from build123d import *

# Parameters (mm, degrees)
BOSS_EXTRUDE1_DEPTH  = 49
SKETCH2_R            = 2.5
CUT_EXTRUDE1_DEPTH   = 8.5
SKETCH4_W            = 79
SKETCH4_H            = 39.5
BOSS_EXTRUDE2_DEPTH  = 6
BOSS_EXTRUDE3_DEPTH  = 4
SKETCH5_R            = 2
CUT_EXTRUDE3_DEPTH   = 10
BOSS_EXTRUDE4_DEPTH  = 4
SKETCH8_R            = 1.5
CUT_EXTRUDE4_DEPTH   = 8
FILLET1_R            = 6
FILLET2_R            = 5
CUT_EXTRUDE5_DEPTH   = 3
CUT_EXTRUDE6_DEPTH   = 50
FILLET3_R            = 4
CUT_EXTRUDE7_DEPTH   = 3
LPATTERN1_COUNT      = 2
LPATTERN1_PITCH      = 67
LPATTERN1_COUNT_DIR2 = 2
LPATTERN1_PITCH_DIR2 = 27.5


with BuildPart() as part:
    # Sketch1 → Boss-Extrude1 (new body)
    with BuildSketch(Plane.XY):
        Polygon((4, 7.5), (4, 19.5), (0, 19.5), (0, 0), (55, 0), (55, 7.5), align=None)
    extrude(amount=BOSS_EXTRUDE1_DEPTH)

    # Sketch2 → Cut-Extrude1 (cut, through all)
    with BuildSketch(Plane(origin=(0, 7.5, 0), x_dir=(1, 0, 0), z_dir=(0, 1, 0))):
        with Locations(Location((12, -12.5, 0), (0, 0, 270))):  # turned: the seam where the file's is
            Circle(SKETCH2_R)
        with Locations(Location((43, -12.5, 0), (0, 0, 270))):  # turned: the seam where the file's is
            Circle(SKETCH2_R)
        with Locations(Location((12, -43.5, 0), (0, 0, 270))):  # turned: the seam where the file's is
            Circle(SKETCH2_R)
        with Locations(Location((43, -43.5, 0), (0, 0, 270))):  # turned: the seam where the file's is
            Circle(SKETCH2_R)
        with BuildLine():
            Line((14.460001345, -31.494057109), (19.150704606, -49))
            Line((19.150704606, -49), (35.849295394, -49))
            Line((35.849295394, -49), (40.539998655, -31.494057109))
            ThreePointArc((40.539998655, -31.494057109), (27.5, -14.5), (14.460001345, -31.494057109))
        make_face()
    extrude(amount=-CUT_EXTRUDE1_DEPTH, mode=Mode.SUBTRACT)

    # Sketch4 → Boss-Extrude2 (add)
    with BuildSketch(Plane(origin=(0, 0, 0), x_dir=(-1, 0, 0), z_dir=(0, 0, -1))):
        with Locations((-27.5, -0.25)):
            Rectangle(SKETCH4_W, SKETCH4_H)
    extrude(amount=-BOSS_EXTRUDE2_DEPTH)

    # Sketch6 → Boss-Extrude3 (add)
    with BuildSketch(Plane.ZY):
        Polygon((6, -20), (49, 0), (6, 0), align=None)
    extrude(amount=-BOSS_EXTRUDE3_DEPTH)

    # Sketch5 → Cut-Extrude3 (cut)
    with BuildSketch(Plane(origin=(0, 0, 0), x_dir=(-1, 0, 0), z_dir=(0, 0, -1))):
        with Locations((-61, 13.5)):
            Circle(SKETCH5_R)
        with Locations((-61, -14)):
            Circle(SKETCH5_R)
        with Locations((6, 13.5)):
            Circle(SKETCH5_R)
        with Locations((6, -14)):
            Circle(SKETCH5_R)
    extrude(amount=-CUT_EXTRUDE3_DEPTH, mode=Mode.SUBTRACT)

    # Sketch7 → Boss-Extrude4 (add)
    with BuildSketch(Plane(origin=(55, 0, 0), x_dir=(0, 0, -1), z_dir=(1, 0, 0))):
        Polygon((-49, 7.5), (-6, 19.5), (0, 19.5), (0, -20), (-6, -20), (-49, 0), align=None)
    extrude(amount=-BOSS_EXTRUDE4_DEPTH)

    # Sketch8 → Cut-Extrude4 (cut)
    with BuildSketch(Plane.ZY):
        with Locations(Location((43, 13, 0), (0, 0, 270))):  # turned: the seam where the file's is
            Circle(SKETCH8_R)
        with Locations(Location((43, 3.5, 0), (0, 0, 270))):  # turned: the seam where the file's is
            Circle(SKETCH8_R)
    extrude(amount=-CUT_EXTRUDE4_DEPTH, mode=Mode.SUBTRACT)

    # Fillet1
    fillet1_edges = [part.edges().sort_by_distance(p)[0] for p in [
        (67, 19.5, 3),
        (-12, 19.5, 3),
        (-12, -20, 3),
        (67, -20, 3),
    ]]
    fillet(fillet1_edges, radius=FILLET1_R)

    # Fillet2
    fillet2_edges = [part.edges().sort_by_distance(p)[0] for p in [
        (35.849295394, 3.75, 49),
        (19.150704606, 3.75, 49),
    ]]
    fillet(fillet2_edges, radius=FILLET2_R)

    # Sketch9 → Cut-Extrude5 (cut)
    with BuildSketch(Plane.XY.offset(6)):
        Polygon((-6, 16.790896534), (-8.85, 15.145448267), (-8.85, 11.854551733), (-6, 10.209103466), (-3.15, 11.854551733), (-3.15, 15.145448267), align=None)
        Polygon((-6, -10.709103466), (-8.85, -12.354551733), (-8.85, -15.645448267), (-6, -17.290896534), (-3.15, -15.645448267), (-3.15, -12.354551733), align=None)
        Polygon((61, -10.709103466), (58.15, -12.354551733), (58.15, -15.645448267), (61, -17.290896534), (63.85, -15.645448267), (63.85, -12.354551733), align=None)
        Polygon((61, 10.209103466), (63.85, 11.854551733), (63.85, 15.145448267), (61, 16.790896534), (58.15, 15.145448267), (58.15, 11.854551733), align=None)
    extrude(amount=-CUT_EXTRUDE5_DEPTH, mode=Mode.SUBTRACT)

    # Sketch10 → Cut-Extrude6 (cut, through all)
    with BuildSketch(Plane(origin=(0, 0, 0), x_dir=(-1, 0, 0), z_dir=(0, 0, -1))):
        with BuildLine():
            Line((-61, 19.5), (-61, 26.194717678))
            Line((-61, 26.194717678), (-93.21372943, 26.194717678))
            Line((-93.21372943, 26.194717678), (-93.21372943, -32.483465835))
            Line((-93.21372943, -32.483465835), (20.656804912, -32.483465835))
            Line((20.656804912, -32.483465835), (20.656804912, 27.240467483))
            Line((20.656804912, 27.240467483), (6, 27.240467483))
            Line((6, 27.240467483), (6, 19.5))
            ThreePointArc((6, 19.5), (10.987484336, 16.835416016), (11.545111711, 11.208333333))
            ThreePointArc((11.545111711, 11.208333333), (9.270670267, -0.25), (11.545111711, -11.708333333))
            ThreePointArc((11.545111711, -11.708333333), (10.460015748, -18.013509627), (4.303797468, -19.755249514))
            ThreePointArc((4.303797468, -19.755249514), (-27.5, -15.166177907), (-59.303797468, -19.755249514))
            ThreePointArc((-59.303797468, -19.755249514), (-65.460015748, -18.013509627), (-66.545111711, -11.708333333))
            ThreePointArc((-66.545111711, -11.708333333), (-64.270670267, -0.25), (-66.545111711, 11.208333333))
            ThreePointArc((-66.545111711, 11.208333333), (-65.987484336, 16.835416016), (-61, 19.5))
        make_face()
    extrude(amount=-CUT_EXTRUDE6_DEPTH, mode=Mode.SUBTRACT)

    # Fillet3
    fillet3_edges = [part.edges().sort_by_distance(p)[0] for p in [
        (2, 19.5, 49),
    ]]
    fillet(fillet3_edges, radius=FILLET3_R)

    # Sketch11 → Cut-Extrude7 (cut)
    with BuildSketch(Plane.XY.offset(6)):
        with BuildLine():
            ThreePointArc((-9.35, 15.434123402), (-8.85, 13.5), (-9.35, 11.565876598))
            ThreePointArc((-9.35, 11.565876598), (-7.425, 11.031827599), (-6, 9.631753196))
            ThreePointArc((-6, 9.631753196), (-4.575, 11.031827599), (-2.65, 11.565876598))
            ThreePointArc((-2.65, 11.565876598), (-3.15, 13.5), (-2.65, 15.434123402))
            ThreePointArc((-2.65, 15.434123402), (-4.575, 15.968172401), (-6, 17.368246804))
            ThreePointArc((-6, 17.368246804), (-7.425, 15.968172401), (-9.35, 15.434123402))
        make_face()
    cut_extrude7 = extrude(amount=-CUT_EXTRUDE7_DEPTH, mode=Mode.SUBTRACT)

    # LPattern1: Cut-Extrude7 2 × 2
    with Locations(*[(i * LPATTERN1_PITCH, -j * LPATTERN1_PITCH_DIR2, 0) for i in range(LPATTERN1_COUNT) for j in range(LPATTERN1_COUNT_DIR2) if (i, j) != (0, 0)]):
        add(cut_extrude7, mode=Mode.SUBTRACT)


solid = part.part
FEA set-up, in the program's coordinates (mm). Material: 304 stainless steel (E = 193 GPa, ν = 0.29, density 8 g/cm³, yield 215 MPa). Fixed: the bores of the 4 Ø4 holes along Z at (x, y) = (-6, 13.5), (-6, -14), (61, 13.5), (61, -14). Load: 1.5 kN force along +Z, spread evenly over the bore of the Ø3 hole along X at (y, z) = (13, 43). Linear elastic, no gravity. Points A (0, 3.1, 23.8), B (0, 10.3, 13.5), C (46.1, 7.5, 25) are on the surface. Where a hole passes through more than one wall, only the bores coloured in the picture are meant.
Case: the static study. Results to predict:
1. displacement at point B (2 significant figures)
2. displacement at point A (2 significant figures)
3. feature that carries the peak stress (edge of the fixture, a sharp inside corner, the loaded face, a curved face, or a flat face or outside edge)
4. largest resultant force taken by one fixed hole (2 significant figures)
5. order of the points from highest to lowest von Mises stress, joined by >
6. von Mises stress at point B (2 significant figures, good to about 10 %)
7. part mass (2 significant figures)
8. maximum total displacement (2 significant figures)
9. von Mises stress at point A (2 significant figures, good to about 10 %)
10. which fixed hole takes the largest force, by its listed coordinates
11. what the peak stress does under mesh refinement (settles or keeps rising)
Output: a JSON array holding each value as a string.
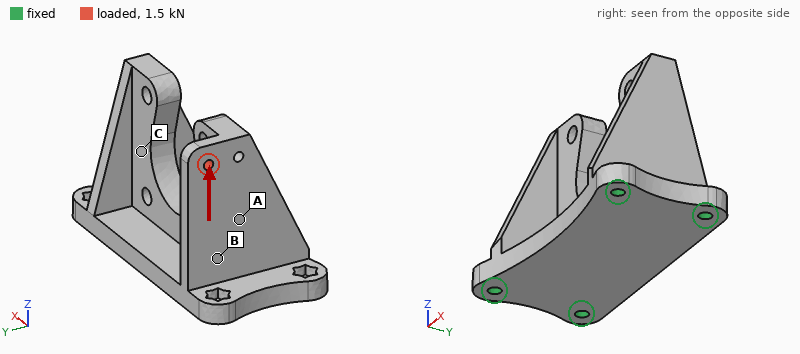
["5.9 µm", "6.3 µm", "edge of the fixture", "1.4 kN", "B > A > C", "25 MPa", "270 g", "18 µm", "11 MPa", "(-6, 13.5)", "keeps rising"]
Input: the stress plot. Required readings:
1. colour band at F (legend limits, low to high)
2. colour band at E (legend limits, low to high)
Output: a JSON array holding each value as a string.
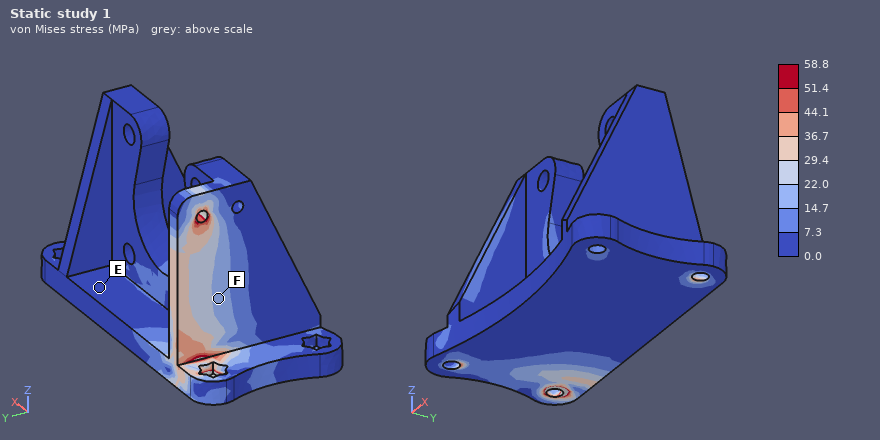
["14.7 to 22.0 MPa", "0.0 to 7.3 MPa"]
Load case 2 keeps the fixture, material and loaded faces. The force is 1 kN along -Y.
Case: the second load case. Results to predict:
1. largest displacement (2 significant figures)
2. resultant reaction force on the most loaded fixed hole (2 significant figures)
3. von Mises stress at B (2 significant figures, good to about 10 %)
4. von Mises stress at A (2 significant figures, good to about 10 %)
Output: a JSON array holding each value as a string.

["34 µm", "1.5 kN", "23 MPa", "17 MPa"]
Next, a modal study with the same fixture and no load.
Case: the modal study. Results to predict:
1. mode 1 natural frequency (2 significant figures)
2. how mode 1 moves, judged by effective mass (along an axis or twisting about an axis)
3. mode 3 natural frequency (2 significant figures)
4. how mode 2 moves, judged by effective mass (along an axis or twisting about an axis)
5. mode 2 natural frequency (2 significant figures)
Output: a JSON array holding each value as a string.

["4600 Hz", "along Z", "6200 Hz", "along Y", "5300 Hz"]
